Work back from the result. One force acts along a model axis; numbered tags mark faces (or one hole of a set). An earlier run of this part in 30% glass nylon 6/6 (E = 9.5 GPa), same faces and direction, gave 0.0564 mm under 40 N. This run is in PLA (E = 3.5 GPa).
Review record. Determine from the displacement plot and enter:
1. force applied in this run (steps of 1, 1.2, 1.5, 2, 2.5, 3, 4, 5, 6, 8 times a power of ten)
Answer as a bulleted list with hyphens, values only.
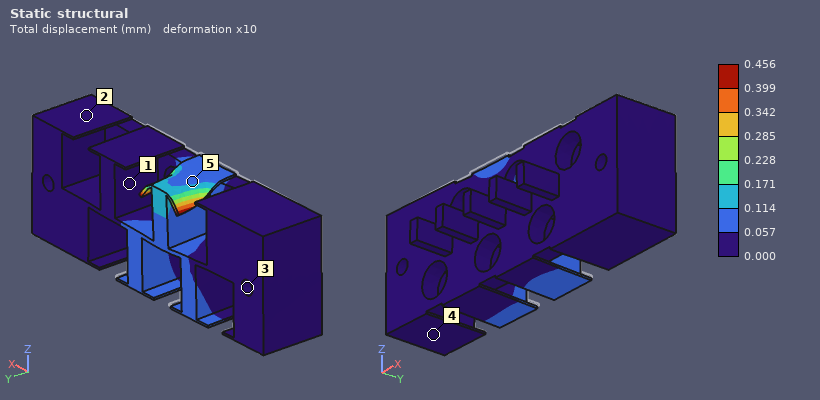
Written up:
- 120 N
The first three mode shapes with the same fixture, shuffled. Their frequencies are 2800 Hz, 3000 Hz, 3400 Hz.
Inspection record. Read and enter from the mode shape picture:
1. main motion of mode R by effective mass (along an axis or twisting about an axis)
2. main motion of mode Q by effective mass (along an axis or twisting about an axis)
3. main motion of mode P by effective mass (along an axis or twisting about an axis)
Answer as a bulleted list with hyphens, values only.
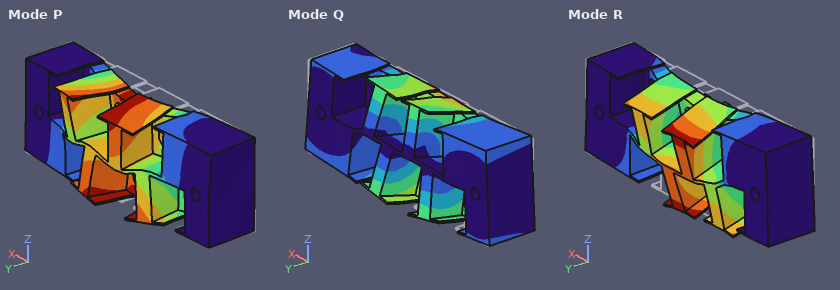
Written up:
- along Z
- along Z
- along Y
